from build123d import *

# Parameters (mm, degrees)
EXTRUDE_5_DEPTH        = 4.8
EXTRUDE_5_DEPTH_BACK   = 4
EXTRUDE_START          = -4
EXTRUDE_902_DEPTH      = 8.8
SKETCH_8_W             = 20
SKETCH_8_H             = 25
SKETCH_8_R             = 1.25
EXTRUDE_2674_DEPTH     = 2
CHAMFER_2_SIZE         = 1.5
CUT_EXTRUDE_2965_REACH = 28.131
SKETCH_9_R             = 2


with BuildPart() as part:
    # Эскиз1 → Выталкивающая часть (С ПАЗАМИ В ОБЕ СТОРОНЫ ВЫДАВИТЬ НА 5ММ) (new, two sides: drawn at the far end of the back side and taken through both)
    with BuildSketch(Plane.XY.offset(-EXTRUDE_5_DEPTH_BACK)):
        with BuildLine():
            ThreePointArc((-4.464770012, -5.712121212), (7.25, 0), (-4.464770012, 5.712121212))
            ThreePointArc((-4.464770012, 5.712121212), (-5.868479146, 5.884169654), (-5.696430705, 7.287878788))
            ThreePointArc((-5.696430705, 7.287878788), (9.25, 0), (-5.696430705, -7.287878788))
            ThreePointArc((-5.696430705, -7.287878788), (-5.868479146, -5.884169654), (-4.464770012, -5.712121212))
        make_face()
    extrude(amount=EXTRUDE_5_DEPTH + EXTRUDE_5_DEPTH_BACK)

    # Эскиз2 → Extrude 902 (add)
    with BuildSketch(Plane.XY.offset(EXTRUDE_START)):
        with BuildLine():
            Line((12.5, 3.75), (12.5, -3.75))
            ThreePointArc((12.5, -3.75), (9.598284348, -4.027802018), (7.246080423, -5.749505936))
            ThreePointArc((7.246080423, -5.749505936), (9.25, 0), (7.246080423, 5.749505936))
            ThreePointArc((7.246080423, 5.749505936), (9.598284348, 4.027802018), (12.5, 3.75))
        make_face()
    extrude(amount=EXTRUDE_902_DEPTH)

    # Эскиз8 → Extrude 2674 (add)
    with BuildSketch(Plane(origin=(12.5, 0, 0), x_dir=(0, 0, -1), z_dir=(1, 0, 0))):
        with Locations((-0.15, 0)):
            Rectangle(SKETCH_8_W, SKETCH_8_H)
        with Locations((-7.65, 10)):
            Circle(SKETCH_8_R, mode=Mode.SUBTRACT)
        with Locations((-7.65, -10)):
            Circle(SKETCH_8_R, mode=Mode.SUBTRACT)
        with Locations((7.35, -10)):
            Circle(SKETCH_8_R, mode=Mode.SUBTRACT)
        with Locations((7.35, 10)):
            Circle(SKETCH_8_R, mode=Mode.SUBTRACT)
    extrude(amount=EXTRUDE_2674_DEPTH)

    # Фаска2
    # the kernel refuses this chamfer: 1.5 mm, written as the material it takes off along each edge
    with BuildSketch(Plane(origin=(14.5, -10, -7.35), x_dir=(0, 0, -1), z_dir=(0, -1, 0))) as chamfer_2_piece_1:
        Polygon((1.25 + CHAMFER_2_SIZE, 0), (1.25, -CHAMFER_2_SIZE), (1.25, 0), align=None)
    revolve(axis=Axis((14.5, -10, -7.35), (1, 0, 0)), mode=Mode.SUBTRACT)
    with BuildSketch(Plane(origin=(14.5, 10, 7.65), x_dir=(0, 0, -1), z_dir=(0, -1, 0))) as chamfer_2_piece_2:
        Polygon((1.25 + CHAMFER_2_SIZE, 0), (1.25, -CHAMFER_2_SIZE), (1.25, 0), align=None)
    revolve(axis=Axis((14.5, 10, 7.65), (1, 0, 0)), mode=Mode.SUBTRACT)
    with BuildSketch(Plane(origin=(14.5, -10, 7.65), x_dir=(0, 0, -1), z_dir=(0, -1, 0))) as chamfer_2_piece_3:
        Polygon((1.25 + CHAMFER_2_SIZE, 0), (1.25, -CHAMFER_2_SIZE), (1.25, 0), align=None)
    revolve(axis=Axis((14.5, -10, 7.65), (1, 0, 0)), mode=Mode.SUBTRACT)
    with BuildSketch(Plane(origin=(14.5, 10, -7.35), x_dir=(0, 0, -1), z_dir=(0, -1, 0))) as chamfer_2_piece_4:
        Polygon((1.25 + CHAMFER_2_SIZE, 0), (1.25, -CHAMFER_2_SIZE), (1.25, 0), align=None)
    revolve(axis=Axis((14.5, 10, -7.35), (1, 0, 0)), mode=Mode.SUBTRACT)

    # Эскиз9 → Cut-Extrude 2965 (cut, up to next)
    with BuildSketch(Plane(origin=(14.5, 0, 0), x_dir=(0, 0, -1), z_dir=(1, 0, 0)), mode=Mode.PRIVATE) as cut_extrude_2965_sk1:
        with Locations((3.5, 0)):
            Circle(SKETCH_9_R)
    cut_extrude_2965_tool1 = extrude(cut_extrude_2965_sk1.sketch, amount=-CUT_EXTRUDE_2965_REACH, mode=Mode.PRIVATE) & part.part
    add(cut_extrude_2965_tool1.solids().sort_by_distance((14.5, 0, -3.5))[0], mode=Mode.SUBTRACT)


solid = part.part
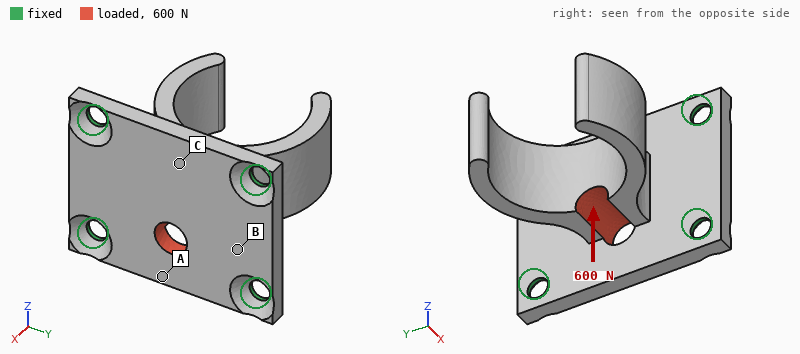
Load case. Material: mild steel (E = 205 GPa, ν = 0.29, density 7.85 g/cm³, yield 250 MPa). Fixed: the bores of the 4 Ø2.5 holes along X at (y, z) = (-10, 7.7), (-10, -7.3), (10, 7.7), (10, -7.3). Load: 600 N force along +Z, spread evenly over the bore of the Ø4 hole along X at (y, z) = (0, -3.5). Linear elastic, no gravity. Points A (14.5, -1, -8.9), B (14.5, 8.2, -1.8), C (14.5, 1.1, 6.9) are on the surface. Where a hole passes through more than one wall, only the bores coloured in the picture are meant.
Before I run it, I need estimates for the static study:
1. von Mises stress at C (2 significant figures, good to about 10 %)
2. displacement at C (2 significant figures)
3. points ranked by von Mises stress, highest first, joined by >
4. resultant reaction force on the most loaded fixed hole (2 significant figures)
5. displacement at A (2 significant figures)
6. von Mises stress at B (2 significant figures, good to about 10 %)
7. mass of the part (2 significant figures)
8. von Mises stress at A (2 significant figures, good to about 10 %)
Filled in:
28 MPa
3.5 µm
A > C > B
160 N
3.9 µm
12 MPa
14 g
43 MPa
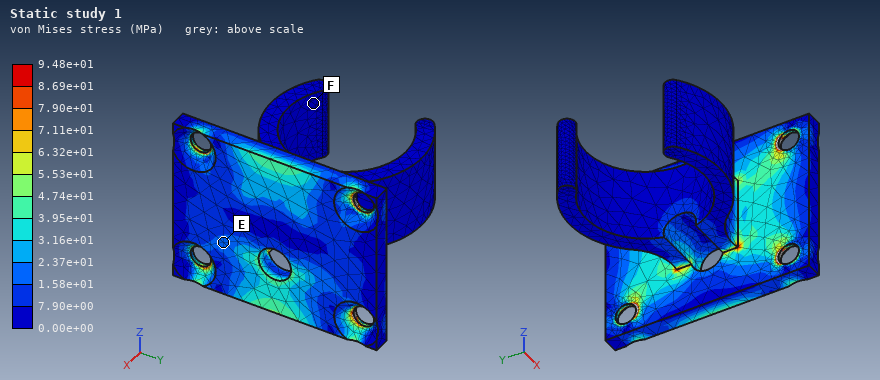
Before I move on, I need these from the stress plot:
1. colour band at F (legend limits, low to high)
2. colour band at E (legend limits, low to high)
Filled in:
0.00e+00 to 7.90e+00 MPa
1.58e+01 to 2.37e+01 MPa
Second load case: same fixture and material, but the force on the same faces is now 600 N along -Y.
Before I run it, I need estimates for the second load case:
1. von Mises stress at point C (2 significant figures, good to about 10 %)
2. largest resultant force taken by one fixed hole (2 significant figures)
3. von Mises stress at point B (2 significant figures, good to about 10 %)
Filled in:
14 MPa
180 N
15 MPa
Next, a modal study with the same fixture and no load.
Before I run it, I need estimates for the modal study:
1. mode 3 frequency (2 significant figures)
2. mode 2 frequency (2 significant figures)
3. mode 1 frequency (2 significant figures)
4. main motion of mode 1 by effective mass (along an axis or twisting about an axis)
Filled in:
7000 Hz
6800 Hz
5300 Hz
along Y
